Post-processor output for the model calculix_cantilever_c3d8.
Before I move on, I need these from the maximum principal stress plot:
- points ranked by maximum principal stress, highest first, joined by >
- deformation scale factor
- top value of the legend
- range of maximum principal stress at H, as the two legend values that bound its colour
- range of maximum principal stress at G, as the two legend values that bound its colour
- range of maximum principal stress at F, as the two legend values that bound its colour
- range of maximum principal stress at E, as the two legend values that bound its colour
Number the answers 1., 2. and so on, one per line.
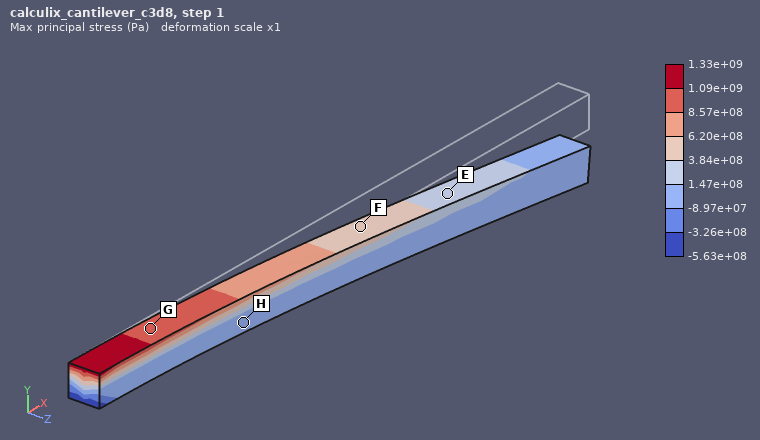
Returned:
1. G > F > E > H
2. 1
3. 1.33e+09 Pa
4. -8.97e+07 to 1.47e+08 Pa
5. 8.57e+08 to 1.09e+09 Pa
6. 3.84e+08 to 6.20e+08 Pa
7. 1.47e+08 to 3.84e+08 Pa
